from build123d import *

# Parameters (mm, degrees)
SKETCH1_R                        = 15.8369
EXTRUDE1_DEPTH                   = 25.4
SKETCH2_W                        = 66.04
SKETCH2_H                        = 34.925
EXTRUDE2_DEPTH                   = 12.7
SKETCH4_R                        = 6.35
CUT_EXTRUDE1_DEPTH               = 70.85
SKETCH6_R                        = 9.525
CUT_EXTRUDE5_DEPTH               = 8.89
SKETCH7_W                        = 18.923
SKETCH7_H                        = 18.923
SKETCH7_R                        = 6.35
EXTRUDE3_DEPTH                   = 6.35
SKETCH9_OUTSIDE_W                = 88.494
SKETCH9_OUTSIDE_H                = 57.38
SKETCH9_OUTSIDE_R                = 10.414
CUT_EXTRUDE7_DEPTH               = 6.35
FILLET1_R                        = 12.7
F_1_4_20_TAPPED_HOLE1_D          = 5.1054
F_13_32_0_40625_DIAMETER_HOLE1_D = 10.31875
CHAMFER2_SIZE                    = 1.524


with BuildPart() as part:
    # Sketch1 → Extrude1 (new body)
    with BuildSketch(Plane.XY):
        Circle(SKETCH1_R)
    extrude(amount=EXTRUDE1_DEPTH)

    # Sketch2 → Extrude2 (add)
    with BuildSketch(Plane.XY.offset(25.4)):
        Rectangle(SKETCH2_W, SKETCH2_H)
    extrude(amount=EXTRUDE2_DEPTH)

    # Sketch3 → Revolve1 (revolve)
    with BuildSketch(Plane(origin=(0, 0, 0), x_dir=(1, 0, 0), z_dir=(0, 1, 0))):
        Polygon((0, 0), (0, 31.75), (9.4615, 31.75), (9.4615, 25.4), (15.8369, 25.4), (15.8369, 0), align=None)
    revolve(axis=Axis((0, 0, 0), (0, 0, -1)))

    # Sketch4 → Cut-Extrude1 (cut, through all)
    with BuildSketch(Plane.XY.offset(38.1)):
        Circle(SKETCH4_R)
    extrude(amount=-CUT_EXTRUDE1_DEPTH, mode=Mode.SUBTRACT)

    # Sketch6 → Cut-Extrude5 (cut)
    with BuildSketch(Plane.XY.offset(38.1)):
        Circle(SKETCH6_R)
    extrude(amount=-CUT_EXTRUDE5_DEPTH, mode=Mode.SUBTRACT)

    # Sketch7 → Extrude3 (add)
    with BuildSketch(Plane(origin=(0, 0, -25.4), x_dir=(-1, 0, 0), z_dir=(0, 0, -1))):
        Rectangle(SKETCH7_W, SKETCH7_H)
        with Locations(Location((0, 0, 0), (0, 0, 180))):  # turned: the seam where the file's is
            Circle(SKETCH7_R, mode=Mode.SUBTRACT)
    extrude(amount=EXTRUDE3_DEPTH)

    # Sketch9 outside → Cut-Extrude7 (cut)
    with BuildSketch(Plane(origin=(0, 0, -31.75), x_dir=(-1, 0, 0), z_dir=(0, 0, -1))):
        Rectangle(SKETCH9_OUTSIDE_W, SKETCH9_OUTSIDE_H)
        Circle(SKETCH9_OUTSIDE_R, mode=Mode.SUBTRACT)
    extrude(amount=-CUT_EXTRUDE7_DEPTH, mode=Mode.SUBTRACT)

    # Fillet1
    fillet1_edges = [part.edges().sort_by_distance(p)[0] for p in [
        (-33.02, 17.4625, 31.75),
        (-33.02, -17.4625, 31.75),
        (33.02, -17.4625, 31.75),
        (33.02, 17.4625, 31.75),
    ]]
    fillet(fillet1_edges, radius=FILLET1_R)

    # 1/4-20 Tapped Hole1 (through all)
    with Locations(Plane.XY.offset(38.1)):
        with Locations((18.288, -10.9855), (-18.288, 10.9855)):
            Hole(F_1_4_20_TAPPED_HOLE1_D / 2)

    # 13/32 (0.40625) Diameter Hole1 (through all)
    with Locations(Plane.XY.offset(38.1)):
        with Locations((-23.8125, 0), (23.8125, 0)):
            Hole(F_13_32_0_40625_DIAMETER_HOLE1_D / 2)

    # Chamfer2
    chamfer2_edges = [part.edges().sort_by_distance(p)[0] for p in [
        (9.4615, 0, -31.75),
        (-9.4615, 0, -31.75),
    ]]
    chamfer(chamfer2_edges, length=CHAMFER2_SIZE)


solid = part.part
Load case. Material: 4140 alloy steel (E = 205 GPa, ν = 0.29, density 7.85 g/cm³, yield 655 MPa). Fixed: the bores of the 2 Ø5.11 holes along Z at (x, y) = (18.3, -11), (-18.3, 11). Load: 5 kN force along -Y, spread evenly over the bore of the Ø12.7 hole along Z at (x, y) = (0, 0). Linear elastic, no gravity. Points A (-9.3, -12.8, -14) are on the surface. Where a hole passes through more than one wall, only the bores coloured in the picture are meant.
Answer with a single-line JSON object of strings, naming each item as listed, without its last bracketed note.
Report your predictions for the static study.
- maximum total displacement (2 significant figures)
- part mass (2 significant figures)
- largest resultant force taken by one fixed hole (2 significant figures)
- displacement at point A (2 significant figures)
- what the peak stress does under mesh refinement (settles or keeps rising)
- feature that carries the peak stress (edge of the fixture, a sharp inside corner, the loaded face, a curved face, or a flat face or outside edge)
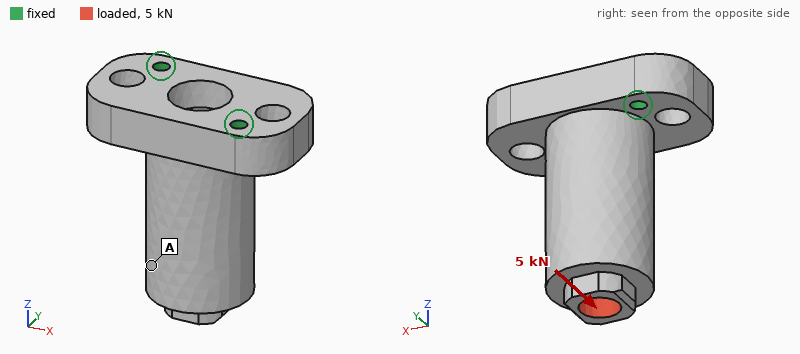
{"maximum total displacement": "83 µm", "part mass": "440 g", "largest resultant force taken by one fixed hole": "3.5 kN", "displacement at point A": "62 µm", "what the peak stress does under mesh refinement": "keeps rising", "feature that carries the peak stress": "edge of the fixture"}
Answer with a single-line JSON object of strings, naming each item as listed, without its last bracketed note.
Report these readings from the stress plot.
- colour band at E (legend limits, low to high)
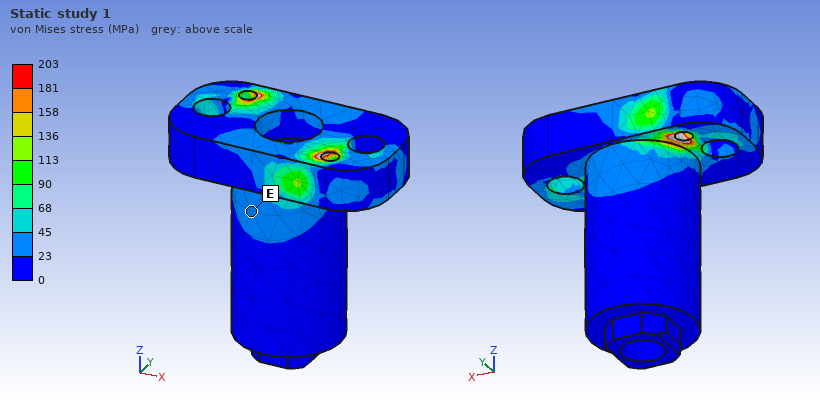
{"colour band at E": "23 to 45 MPa"}
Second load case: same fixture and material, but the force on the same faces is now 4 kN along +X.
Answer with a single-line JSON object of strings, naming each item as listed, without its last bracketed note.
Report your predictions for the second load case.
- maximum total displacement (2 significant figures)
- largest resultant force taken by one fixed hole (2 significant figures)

{"maximum total displacement": "42 µm", "largest resultant force taken by one fixed hole": "3.6 kN"}
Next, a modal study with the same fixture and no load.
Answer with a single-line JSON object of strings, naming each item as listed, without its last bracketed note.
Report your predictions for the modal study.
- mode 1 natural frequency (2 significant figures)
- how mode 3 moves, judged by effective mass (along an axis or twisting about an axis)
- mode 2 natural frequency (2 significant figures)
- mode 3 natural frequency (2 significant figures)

{"mode 1 natural frequency": "2700 Hz", "how mode 3 moves, judged by effective mass": "along Z", "mode 2 natural frequency": "5200 Hz", "mode 3 natural frequency": "11 kHz"}
